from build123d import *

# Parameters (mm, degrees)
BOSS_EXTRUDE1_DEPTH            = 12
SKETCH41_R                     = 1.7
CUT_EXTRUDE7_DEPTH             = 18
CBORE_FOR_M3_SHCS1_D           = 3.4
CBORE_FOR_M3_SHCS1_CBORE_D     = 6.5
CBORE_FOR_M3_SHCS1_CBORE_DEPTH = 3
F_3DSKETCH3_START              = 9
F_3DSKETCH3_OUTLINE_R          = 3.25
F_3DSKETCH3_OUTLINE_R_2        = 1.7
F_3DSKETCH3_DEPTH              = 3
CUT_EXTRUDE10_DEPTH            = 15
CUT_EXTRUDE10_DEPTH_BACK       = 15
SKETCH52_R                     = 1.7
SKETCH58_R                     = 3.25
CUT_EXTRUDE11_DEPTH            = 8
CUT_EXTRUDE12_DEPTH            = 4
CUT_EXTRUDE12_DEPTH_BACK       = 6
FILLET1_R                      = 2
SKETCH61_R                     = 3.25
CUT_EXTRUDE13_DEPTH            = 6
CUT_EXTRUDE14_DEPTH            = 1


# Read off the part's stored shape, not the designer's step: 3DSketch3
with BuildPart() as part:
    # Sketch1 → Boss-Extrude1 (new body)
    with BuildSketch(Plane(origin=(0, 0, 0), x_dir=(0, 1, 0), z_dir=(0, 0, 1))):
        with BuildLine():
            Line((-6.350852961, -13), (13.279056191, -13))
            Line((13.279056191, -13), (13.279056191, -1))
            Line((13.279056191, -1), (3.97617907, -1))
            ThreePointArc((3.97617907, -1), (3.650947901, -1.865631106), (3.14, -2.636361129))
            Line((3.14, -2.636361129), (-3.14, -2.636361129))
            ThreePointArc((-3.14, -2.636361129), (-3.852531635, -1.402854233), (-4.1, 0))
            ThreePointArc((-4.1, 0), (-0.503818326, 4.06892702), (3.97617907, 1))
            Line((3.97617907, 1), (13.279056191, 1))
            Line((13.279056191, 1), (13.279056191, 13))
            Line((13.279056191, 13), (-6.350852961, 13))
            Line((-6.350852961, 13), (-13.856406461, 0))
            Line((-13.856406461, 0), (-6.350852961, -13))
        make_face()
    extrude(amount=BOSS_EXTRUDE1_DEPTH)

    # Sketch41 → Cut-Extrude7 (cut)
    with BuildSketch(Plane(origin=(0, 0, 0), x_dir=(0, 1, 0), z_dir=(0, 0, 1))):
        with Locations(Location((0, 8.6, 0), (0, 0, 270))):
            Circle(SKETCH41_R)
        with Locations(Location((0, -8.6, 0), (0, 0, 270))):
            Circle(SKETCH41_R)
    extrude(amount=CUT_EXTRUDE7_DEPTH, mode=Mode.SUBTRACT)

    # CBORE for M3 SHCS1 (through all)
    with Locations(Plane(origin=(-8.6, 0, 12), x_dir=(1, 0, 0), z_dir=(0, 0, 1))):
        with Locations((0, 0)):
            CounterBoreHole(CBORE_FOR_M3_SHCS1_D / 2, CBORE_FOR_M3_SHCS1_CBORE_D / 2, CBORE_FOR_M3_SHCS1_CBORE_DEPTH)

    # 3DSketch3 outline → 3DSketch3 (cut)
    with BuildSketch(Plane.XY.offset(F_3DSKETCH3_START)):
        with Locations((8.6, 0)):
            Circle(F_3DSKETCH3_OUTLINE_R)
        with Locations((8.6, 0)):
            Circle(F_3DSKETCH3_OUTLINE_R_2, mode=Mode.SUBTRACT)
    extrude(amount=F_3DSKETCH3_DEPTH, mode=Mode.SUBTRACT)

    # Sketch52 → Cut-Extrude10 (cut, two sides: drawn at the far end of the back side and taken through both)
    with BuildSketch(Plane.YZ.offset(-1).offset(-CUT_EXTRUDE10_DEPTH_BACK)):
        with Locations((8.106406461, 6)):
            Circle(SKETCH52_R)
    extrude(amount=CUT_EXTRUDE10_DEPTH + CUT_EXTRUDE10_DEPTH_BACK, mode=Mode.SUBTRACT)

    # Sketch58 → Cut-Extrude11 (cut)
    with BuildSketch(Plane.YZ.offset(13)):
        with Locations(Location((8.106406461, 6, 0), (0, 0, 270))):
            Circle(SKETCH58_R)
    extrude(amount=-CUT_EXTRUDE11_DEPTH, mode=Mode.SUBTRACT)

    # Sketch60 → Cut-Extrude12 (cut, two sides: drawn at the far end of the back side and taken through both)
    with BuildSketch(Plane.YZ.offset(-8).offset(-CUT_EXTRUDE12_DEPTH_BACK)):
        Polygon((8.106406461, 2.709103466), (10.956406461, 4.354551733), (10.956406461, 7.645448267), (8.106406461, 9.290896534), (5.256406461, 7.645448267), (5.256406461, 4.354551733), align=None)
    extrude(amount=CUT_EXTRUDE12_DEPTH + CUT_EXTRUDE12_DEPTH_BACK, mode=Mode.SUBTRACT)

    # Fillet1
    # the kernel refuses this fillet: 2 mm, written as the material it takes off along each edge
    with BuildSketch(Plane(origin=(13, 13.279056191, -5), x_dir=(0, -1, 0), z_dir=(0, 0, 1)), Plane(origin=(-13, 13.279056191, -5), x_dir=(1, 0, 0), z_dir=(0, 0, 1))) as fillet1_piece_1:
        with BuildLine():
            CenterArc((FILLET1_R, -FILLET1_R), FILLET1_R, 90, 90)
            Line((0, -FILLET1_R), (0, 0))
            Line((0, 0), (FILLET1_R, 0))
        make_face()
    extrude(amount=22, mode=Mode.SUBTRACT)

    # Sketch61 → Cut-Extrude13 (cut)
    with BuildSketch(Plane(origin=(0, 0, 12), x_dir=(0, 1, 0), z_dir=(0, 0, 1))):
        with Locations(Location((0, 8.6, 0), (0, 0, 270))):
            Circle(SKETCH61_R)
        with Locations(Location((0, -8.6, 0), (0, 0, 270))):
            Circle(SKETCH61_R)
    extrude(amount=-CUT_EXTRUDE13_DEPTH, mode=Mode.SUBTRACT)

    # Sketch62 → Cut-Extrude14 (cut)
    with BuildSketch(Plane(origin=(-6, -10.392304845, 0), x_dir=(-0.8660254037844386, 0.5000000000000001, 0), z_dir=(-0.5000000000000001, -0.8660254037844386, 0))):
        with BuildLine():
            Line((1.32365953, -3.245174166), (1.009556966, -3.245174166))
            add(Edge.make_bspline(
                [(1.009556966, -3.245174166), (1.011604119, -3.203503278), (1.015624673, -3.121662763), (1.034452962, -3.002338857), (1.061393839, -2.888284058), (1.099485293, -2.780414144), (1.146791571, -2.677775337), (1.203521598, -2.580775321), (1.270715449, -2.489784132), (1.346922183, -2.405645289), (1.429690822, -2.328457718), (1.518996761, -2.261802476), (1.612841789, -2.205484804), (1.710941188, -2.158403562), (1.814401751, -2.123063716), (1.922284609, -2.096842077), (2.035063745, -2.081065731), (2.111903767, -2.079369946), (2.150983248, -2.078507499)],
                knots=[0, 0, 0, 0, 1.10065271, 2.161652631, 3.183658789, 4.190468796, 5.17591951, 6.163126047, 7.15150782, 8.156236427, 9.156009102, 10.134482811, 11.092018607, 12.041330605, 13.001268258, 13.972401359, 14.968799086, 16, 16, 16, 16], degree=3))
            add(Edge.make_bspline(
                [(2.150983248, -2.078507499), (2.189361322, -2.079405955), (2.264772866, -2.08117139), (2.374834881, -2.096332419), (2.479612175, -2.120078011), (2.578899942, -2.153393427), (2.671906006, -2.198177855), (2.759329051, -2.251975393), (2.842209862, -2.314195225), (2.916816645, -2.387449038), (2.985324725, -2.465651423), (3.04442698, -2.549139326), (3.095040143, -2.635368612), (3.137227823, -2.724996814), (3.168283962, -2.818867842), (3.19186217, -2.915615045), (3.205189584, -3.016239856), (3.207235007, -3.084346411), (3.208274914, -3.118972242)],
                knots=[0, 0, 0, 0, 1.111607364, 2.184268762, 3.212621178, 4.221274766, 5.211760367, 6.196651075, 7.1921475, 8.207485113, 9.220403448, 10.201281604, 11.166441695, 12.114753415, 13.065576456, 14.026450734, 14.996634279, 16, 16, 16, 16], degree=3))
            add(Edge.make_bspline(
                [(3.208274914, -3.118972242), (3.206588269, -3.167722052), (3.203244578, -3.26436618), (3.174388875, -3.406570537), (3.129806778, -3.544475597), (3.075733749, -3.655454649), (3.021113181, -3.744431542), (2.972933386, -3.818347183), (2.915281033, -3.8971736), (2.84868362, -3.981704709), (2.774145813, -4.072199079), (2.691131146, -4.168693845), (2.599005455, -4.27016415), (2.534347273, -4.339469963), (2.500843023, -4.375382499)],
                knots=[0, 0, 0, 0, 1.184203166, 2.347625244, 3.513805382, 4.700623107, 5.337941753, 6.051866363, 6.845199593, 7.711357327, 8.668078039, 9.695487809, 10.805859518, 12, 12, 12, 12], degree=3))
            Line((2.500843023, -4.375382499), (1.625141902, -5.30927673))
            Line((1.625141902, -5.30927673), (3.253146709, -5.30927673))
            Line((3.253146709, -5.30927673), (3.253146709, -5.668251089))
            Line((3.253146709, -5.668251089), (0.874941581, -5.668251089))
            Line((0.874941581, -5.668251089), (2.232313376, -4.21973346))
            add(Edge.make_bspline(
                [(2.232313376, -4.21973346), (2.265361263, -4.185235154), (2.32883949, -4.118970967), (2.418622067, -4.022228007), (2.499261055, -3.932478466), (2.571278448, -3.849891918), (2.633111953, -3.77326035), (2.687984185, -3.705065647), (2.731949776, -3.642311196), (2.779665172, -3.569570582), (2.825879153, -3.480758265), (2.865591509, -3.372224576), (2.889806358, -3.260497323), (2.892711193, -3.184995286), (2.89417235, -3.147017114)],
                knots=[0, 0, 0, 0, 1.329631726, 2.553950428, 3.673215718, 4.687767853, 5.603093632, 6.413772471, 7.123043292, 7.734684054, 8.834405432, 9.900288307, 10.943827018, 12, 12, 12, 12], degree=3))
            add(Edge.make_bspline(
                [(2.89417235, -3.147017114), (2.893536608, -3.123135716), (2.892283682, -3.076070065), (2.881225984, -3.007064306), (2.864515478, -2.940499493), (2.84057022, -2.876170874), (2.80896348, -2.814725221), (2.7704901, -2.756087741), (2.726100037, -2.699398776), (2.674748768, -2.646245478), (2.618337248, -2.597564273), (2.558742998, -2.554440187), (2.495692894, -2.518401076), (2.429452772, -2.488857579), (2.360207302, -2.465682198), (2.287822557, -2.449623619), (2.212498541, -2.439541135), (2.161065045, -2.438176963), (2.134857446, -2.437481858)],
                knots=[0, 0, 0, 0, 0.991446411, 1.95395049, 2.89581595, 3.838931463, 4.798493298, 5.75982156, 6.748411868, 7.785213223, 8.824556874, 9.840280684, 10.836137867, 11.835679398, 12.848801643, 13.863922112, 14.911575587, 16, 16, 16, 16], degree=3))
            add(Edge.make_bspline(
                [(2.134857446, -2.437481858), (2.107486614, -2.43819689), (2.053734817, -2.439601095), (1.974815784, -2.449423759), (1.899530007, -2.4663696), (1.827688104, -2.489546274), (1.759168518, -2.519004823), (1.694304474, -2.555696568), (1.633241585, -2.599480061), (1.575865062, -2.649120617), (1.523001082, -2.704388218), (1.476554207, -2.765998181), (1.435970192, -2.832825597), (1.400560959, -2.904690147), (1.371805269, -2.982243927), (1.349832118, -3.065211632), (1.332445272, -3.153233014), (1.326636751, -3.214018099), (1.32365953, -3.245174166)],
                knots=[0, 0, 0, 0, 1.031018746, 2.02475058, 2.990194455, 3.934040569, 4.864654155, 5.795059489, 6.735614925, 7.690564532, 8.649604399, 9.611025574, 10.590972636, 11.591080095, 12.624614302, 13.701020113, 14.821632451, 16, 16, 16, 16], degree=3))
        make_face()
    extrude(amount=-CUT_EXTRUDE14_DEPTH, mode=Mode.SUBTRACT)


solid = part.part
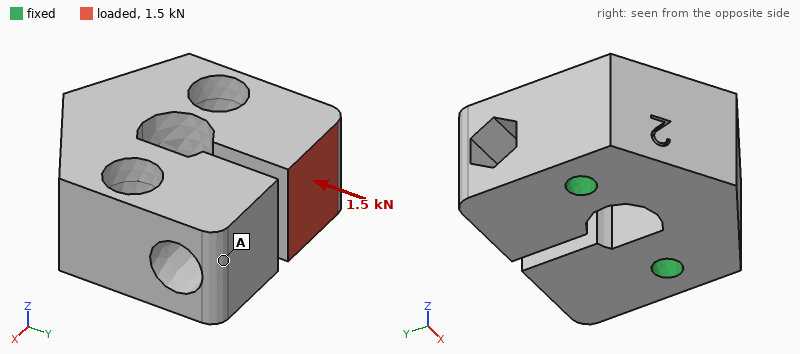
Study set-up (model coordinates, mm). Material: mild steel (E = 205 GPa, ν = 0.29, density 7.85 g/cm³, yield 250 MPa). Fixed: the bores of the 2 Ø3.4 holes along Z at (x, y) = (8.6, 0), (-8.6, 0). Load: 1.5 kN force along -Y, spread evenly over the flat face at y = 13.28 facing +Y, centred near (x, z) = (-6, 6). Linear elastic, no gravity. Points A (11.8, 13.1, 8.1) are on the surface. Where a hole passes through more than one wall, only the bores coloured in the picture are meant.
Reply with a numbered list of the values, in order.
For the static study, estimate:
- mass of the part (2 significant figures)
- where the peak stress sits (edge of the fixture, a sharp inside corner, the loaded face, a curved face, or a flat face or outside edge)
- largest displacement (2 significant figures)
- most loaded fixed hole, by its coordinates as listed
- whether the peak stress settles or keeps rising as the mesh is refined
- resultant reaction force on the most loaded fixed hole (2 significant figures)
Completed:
1. 42 g
2. edge of the fixture
3. 6.2 µm
4. (-8.6, 0)
5. keeps rising
6. 1.4 kN
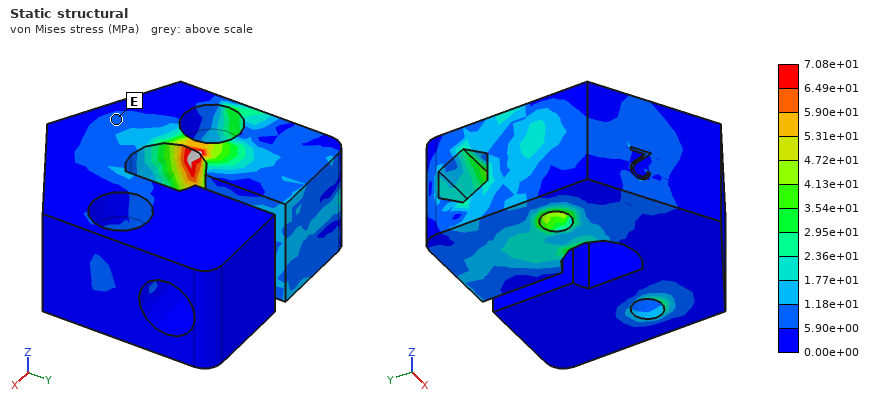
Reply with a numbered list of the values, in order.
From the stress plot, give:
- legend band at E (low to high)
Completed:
1. 5.90e+00 to 1.18e+01 MPa
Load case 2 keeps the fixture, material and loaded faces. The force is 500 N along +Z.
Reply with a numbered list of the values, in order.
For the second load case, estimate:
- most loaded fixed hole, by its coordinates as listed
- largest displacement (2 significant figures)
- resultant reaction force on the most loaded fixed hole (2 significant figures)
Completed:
1. (-8.6, 0)
2. 8.0 µm
3. 520 N
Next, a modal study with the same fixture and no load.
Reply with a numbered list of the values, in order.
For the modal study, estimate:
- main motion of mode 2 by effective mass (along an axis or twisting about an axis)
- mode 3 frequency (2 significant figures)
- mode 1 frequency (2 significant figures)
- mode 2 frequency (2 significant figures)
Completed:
1. along X
2. 21 kHz
3. 17 kHz
4. 20 kHz
